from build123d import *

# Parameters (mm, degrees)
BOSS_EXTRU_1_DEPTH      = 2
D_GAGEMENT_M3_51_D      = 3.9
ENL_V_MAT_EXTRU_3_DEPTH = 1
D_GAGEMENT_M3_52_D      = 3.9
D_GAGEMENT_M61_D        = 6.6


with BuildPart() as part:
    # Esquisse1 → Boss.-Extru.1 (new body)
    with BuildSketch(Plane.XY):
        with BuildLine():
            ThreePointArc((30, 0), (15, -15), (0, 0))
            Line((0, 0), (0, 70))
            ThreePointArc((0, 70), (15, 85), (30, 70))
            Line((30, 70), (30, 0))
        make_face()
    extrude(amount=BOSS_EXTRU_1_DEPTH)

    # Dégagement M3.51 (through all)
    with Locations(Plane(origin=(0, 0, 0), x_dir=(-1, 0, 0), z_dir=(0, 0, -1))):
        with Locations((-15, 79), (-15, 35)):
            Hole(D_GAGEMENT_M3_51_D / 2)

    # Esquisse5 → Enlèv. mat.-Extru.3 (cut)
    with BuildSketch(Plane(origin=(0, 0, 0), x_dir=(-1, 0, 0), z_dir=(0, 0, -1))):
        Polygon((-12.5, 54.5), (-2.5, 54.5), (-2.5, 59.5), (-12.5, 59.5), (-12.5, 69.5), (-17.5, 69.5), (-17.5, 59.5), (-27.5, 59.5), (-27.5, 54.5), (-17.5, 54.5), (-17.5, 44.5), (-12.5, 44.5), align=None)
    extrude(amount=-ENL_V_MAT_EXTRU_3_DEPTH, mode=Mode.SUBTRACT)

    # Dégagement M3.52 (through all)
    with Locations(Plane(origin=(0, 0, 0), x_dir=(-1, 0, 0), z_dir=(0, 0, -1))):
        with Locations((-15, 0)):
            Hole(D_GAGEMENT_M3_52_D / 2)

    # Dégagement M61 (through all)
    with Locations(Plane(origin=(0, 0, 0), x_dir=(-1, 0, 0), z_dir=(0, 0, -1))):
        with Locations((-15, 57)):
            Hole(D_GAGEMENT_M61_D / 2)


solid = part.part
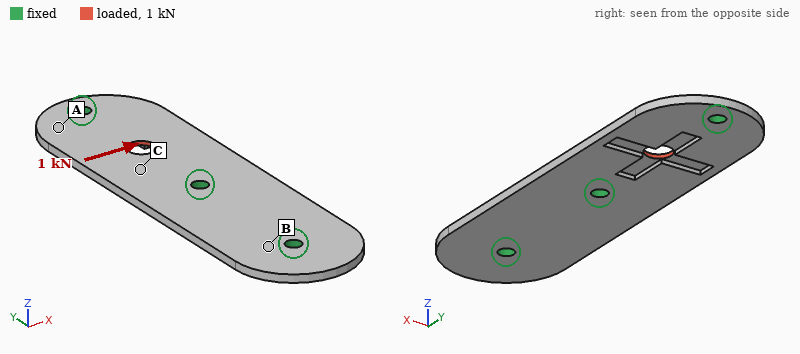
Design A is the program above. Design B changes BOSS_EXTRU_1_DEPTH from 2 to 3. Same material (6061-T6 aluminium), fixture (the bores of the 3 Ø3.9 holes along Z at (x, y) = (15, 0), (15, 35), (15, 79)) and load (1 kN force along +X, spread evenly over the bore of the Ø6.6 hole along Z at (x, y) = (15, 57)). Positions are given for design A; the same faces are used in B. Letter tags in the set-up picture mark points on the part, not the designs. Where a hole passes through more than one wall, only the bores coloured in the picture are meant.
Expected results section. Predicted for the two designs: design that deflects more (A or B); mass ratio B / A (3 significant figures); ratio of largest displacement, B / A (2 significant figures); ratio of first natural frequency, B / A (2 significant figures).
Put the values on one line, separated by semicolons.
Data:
A; 1.52; 0.38; 1.4
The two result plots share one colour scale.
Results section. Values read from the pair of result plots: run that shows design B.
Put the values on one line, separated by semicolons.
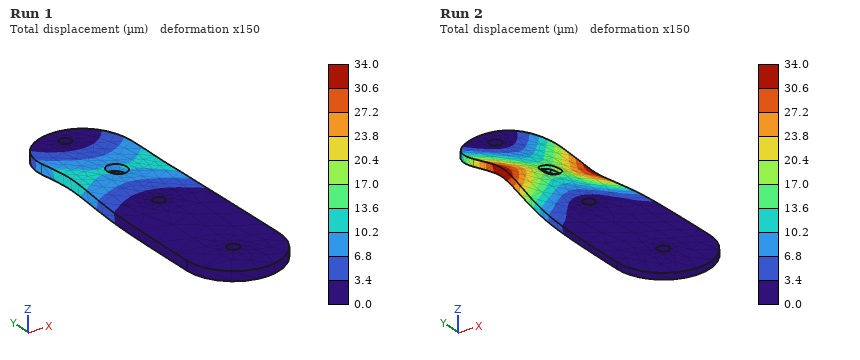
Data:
Run 1
